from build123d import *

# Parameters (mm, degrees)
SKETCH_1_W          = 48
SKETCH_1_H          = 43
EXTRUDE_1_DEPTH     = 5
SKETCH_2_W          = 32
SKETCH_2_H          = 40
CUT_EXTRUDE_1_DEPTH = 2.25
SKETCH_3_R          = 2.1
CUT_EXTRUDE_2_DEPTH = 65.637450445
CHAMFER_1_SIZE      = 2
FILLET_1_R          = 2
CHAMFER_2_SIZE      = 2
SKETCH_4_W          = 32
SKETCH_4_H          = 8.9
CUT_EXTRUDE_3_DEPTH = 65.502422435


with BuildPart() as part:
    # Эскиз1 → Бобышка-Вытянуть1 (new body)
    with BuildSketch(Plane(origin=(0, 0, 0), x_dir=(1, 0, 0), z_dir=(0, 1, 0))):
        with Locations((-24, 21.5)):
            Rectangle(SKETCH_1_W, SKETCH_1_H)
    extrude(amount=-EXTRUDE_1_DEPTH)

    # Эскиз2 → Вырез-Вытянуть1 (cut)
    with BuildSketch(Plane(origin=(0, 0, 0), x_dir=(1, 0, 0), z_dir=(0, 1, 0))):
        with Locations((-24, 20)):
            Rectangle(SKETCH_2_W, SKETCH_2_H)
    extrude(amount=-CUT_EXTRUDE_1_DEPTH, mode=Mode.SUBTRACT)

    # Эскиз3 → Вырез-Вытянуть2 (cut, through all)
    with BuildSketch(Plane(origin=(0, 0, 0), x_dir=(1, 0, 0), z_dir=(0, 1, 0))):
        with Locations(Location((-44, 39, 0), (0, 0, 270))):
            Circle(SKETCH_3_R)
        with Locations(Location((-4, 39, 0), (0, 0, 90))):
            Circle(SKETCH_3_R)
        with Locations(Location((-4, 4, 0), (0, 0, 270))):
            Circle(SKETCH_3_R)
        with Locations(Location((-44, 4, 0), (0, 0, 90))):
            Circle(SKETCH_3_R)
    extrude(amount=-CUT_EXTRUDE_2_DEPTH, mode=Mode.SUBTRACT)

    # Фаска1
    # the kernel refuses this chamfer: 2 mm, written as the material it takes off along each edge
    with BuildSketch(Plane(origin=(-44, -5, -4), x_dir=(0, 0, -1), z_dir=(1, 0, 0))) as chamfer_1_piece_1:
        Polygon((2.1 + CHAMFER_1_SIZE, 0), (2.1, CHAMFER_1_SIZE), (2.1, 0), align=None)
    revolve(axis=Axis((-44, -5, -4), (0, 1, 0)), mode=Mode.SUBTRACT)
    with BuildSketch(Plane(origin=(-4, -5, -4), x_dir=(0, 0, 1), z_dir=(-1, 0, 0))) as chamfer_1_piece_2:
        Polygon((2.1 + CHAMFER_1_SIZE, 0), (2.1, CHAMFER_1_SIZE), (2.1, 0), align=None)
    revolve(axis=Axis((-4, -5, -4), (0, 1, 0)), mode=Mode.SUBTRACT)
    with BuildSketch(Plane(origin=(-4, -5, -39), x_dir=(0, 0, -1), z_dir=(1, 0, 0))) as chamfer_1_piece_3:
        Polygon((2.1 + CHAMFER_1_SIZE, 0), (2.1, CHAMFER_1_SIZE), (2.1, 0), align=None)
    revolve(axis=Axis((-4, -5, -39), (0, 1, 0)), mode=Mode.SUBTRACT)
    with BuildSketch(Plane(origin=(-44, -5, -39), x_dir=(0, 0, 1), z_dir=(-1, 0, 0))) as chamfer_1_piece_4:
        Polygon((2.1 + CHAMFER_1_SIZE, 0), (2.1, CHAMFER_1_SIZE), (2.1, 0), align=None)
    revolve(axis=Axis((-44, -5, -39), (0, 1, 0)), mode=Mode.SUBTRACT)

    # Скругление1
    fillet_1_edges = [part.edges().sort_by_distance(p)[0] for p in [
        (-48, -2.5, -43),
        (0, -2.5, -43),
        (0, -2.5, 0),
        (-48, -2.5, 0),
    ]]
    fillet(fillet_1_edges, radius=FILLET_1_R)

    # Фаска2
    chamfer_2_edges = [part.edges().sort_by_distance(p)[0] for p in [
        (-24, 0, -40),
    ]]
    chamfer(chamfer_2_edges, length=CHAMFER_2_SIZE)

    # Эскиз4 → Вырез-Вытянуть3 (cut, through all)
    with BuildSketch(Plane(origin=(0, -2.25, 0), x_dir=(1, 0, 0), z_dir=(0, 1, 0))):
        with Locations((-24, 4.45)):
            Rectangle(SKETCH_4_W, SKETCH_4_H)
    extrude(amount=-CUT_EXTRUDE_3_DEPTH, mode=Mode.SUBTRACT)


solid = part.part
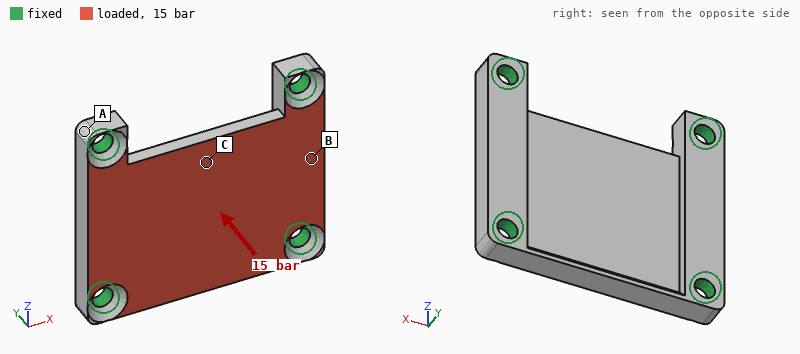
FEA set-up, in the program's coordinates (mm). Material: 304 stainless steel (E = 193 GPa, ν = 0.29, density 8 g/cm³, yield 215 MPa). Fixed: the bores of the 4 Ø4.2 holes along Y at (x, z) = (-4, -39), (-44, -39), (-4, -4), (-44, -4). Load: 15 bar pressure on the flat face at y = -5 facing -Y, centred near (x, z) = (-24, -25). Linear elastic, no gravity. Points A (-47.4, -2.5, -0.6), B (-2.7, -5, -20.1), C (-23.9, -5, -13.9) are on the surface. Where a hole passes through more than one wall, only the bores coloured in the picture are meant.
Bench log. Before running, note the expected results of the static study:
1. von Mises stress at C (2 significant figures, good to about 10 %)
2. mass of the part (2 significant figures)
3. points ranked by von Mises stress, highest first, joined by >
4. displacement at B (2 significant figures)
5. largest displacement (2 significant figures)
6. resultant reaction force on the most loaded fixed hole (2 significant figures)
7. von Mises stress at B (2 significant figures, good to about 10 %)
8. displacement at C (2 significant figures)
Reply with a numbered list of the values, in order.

1. 77 MPa
2. 49 g
3. C > B > A
4. 6.8 µm
5. 35 µm
6. 970 N
7. 40 MPa
8. 34 µm
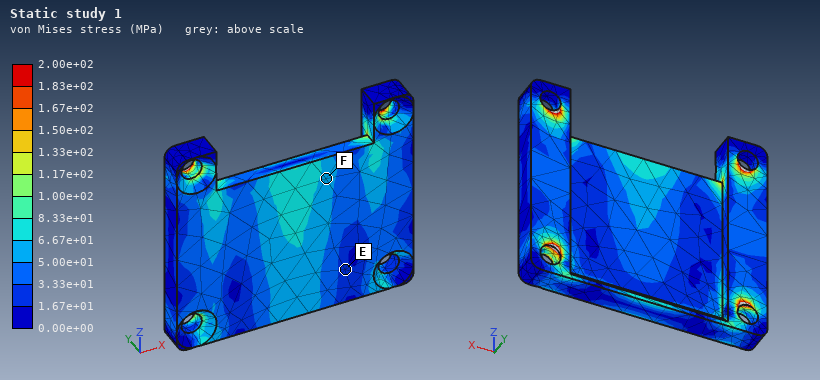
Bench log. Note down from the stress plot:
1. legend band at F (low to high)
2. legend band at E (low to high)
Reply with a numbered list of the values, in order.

1. 5.00e+01 to 6.67e+01 MPa
2. 1.67e+01 to 3.33e+01 MPa
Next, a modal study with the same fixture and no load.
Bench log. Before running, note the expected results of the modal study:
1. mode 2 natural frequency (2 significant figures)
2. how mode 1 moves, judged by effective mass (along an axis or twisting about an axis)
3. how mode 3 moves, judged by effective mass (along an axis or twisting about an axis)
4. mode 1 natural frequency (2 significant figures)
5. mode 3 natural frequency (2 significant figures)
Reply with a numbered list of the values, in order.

1. 13 kHz
2. along Y
3. twisting about Z
4. 8400 Hz
5. 16 kHz
